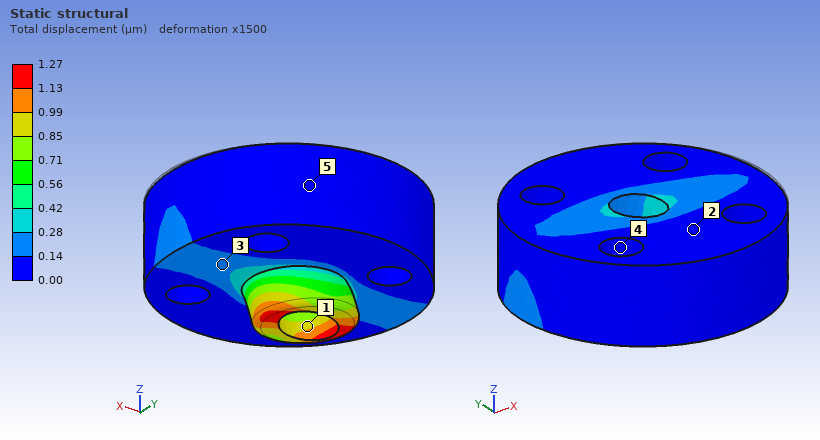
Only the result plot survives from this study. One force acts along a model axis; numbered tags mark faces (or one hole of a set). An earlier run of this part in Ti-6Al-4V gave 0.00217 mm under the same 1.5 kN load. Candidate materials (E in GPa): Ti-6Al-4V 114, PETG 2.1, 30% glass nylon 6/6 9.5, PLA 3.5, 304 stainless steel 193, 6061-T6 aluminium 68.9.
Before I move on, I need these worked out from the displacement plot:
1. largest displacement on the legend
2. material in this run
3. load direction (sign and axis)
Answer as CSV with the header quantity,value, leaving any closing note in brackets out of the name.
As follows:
quantity,value
largest displacement on the legend,1.27 µm
material in this run,304 stainless steel
load direction,-X
